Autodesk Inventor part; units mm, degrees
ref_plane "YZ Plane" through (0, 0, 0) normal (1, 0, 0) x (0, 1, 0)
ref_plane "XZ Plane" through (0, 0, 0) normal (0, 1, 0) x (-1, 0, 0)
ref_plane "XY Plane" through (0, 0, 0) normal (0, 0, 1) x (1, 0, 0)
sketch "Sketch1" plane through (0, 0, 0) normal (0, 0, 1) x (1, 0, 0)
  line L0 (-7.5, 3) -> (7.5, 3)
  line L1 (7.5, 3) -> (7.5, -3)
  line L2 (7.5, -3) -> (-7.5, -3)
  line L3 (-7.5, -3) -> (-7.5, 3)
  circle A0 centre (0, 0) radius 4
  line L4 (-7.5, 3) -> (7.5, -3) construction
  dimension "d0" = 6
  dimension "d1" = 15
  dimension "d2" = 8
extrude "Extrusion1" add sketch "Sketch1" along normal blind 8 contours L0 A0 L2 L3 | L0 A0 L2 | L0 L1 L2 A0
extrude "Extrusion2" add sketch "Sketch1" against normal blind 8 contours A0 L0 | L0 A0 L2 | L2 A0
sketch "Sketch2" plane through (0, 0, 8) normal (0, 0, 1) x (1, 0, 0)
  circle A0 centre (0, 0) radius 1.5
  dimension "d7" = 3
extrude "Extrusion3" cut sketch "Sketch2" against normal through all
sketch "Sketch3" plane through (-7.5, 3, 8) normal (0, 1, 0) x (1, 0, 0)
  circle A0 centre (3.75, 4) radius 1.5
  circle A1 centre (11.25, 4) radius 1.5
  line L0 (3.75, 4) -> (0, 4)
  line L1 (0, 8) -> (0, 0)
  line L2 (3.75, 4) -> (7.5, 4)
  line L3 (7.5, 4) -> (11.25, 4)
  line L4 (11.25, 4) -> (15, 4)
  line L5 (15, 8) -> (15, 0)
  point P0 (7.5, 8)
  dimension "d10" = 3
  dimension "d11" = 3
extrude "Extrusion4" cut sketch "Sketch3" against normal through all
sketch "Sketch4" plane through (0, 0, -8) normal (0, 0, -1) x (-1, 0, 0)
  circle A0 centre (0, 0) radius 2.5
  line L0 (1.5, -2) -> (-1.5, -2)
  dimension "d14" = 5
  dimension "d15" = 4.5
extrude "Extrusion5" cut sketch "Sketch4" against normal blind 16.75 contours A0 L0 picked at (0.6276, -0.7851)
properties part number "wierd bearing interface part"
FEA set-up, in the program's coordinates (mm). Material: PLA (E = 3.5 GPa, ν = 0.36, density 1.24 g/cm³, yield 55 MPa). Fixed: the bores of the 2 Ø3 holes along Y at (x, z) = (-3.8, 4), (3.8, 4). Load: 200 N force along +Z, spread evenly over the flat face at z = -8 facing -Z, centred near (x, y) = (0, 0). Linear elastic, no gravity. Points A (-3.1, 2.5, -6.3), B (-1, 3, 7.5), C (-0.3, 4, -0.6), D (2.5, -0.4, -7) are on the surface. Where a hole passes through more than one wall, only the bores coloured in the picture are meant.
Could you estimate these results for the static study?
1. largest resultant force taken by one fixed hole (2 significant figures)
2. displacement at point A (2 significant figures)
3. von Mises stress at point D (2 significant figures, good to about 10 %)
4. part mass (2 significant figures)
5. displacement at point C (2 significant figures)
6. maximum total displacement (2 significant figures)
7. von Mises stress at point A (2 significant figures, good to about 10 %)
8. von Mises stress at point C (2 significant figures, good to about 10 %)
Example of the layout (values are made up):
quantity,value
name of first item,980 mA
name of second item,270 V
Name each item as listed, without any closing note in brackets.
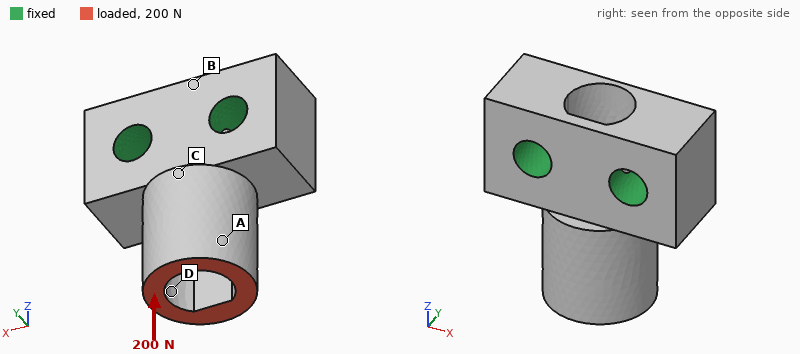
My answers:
quantity,value
largest resultant force taken by one fixed hole,100 N
displacement at point A,18 µm
von Mises stress at point D,7.1 MPa
part mass,0.92 g
displacement at point C,12 µm
maximum total displacement,21 µm
von Mises stress at point A,6.3 MPa
von Mises stress at point C,1.9 MPa
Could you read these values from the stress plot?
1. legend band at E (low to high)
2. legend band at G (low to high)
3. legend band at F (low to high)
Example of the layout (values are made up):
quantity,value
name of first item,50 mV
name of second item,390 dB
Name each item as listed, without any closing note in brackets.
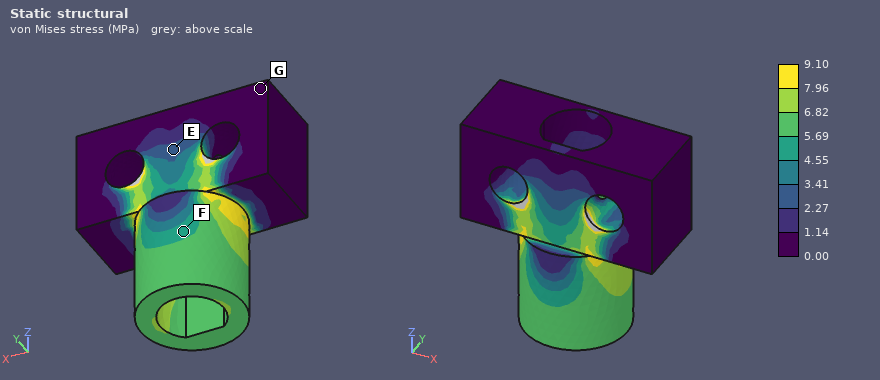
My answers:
quantity,value
legend band at E,2.27 to 3.41 MPa
legend band at G,0.00 to 1.14 MPa
legend band at F,4.55 to 5.69 MPa
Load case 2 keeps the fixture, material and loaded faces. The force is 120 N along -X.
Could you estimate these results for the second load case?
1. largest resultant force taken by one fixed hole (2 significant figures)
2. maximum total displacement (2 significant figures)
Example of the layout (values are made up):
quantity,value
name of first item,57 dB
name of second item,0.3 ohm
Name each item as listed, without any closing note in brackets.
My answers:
quantity,value
largest resultant force taken by one fixed hole,170 N
maximum total displacement,0.12 mm
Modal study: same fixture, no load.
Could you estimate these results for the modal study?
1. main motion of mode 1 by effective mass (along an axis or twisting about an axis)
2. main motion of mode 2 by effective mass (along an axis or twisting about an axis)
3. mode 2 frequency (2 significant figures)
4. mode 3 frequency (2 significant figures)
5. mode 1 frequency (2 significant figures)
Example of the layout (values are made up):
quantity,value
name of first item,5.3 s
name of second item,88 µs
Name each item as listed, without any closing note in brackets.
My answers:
quantity,value
main motion of mode 1 by effective mass,along Y
main motion of mode 2 by effective mass,along X
mode 2 frequency,16 kHz
mode 3 frequency,24 kHz
mode 1 frequency,11 kHz
